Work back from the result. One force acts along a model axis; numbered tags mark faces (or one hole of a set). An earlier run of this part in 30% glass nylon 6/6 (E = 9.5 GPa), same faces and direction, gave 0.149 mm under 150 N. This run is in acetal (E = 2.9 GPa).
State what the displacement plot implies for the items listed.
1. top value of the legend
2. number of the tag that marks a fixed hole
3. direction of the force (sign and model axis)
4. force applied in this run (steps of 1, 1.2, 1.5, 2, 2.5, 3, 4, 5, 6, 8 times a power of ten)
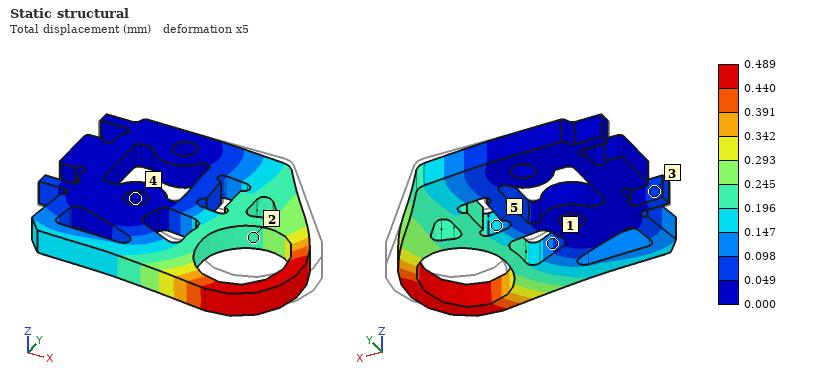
0.489 mm
4
-Y
150 N
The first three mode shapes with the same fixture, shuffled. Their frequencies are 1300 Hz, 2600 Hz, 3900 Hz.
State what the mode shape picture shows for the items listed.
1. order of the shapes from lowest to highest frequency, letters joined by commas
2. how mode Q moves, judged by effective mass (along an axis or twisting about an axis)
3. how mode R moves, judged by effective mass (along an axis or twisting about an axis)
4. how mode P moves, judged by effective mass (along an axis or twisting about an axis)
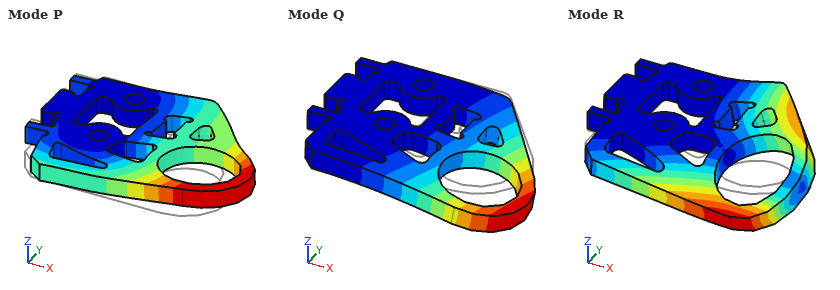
Q, R, P
along Z
twisting about X
along Y
